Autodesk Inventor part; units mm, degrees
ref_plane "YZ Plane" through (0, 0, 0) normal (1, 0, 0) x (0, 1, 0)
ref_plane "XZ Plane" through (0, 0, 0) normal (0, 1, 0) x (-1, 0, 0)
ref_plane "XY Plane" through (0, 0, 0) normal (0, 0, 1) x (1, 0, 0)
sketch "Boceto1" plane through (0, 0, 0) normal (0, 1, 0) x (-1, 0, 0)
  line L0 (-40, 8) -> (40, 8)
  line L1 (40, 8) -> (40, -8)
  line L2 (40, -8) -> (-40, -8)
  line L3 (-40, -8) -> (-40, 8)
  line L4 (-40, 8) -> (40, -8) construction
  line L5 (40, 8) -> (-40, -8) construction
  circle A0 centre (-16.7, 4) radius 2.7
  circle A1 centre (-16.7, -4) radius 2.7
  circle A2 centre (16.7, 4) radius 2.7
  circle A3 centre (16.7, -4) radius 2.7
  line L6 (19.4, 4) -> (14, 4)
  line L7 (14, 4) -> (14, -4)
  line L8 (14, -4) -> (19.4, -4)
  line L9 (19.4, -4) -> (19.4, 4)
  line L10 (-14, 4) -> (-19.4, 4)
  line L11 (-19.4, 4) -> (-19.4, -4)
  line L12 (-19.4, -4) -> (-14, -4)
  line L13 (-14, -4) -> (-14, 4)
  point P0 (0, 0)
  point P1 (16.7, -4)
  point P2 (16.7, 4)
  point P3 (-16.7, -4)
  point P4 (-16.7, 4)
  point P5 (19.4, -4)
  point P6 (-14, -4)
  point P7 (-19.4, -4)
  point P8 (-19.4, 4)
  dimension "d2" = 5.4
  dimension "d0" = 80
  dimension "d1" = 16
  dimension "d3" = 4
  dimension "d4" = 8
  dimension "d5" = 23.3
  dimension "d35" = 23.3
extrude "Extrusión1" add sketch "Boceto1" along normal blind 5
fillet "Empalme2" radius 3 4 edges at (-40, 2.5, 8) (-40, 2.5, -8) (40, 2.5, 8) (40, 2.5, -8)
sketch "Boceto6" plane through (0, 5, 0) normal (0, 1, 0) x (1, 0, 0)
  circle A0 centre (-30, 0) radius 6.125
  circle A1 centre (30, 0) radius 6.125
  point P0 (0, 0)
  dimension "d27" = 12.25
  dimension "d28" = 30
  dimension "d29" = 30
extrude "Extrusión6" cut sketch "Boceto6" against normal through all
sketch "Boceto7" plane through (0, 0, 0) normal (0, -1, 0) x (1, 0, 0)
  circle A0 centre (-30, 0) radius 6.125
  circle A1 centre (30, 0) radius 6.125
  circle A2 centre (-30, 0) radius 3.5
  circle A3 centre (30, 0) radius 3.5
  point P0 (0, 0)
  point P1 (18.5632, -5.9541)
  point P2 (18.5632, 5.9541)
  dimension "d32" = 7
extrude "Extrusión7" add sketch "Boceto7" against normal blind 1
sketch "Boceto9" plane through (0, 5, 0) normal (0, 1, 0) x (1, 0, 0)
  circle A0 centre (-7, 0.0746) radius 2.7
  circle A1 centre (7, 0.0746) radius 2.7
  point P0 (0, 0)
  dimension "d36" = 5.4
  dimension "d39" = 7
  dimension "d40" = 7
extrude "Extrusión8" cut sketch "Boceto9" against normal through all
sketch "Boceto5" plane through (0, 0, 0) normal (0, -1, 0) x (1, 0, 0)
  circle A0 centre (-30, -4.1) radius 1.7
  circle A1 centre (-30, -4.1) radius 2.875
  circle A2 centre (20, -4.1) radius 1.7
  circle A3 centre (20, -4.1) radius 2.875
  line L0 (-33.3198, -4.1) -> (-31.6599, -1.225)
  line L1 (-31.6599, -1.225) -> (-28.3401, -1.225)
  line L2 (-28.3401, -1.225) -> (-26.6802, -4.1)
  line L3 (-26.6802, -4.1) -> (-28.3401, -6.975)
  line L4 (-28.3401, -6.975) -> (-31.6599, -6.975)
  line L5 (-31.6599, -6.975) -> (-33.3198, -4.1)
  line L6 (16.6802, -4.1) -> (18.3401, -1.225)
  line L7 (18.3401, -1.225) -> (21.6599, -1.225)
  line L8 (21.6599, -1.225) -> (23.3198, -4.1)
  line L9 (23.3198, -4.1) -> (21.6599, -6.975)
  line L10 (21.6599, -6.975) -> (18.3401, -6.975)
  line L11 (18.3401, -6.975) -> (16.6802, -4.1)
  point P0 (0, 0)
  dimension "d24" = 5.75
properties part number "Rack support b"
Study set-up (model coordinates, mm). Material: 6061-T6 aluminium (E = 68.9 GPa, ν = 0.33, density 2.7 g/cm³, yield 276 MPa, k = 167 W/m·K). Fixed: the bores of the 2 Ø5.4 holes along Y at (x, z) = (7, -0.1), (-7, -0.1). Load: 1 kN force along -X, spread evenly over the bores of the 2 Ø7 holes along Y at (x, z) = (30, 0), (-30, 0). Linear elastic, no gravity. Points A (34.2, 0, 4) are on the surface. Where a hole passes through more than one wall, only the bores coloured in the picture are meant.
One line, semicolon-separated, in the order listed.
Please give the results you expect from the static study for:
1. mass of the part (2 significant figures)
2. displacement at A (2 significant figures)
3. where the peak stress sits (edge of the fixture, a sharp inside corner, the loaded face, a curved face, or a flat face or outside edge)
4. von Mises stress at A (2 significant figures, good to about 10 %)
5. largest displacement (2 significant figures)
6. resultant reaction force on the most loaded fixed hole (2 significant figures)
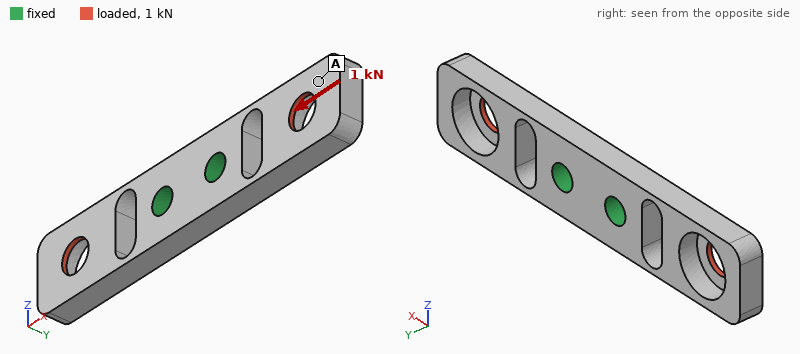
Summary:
12 g; 0.090 mm; a curved face; 17 MPa; 0.12 mm; 500 N
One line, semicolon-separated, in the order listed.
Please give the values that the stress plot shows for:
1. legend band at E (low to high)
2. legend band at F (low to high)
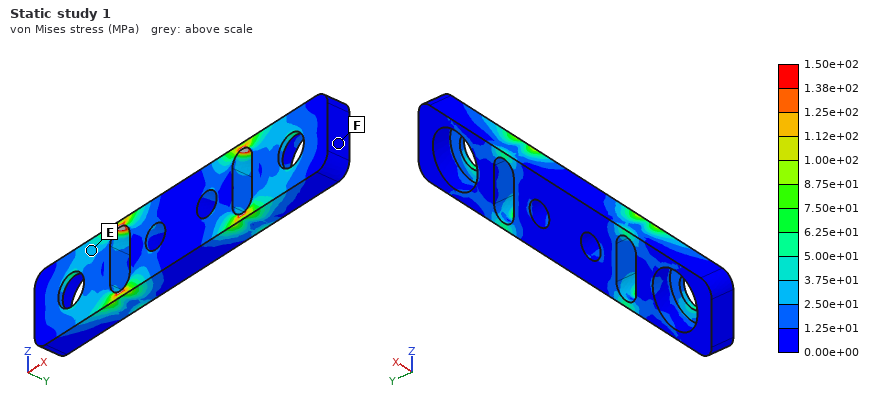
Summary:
2.50e+01 to 3.75e+01 MPa; 0.00e+00 to 1.25e+01 MPa
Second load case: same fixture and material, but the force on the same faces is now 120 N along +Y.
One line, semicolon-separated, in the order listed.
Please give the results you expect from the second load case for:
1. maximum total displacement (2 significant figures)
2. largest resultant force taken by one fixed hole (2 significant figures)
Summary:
100 µm; 60 N
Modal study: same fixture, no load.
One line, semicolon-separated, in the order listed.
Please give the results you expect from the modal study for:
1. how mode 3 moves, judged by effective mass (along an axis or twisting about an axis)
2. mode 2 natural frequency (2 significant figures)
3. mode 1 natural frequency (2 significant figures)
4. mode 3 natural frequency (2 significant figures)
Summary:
twisting about Y; 2700 Hz; 2700 Hz; 6700 Hz
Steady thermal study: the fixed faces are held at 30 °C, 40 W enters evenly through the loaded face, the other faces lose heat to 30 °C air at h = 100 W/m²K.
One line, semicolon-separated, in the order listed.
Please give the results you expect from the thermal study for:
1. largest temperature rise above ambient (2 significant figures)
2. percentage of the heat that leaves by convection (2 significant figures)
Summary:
77 K; 33 %
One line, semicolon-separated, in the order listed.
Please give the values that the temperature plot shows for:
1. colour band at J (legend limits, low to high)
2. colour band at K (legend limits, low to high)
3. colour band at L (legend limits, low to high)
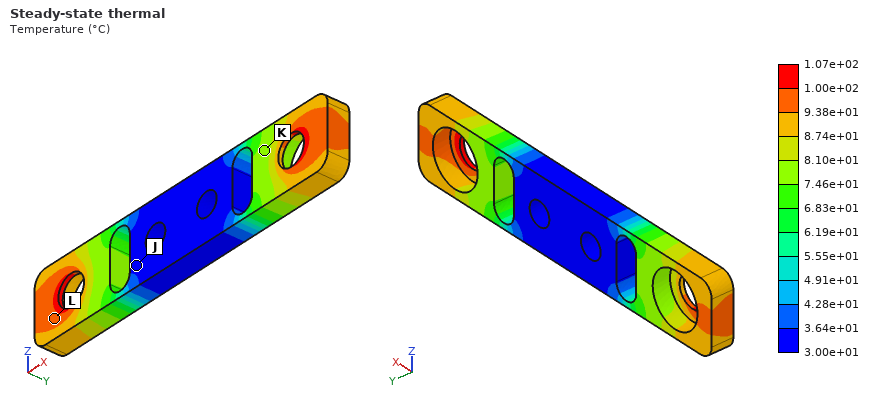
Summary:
3.00e+01 to 3.64e+01 °C; 7.46e+01 to 8.10e+01 °C; 9.38e+01 to 1.00e+02 °C
